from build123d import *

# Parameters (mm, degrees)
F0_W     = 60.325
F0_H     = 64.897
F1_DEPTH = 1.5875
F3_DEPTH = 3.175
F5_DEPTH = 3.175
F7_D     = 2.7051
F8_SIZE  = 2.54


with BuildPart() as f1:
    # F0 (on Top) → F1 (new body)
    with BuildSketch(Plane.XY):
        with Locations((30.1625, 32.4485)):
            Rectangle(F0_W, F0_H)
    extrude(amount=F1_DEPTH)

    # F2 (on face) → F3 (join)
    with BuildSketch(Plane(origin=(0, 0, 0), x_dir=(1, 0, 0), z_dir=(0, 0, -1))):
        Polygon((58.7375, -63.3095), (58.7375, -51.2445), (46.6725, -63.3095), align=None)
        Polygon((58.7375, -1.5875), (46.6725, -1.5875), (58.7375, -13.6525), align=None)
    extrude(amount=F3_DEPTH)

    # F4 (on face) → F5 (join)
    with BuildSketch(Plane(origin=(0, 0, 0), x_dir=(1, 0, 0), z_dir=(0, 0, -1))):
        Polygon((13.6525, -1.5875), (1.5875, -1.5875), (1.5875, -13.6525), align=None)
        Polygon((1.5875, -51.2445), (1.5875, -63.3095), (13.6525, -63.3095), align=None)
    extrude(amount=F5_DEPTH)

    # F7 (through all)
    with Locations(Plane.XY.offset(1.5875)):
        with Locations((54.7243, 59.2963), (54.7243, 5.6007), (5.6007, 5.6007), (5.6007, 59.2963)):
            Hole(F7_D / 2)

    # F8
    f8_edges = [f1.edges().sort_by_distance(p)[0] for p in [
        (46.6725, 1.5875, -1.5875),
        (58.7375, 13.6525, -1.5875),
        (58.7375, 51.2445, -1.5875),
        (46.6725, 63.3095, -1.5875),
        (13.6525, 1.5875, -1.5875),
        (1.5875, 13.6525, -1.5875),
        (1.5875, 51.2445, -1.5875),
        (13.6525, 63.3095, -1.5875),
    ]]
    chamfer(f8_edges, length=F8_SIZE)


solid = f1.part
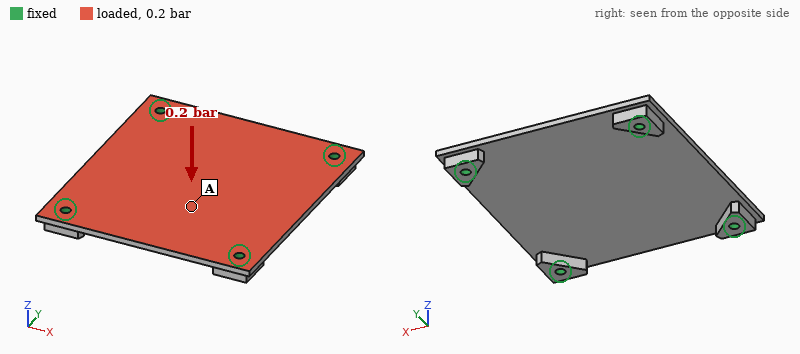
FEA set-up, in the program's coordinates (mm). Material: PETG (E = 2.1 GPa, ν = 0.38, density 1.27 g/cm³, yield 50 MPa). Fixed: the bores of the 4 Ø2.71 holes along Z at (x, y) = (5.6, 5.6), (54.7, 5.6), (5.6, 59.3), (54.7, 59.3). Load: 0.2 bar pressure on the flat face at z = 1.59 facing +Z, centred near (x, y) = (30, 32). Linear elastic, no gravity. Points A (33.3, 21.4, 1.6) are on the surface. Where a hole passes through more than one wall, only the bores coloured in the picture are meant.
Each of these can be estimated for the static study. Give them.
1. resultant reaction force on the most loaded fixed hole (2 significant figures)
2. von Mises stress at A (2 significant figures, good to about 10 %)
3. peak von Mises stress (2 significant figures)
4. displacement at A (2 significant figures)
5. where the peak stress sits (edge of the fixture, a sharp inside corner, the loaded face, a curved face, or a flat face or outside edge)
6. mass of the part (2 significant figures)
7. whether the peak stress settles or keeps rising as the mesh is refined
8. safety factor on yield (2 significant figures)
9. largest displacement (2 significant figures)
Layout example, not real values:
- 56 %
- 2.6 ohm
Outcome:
- 23 N
- 5.2 MPa
- 15 MPa
- 0.79 mm
- the loaded face
- 8.9 g
- settles
- 3.3
- 0.94 mm
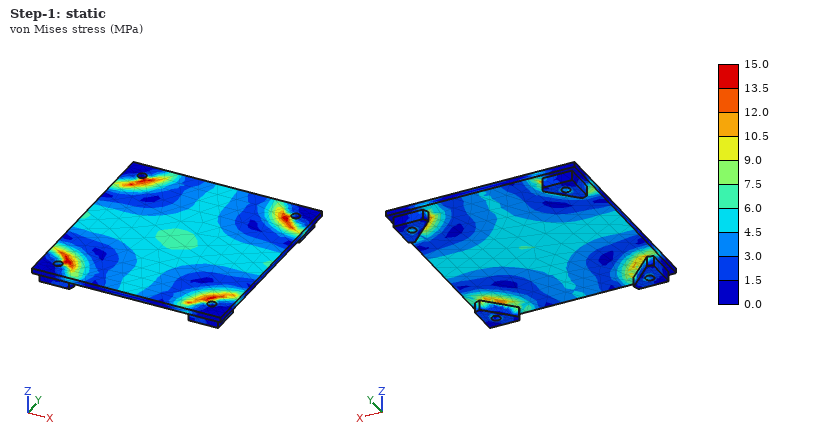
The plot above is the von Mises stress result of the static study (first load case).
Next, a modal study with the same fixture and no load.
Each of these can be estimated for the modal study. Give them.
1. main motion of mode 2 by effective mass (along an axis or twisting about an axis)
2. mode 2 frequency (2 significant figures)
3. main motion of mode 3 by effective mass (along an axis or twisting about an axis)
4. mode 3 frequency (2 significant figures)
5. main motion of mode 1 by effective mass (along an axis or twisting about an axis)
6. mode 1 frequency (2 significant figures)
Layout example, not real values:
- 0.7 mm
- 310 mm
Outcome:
- twisting about Y
- 1100 Hz
- twisting about X
- 1200 Hz
- along Z
- 640 Hz
